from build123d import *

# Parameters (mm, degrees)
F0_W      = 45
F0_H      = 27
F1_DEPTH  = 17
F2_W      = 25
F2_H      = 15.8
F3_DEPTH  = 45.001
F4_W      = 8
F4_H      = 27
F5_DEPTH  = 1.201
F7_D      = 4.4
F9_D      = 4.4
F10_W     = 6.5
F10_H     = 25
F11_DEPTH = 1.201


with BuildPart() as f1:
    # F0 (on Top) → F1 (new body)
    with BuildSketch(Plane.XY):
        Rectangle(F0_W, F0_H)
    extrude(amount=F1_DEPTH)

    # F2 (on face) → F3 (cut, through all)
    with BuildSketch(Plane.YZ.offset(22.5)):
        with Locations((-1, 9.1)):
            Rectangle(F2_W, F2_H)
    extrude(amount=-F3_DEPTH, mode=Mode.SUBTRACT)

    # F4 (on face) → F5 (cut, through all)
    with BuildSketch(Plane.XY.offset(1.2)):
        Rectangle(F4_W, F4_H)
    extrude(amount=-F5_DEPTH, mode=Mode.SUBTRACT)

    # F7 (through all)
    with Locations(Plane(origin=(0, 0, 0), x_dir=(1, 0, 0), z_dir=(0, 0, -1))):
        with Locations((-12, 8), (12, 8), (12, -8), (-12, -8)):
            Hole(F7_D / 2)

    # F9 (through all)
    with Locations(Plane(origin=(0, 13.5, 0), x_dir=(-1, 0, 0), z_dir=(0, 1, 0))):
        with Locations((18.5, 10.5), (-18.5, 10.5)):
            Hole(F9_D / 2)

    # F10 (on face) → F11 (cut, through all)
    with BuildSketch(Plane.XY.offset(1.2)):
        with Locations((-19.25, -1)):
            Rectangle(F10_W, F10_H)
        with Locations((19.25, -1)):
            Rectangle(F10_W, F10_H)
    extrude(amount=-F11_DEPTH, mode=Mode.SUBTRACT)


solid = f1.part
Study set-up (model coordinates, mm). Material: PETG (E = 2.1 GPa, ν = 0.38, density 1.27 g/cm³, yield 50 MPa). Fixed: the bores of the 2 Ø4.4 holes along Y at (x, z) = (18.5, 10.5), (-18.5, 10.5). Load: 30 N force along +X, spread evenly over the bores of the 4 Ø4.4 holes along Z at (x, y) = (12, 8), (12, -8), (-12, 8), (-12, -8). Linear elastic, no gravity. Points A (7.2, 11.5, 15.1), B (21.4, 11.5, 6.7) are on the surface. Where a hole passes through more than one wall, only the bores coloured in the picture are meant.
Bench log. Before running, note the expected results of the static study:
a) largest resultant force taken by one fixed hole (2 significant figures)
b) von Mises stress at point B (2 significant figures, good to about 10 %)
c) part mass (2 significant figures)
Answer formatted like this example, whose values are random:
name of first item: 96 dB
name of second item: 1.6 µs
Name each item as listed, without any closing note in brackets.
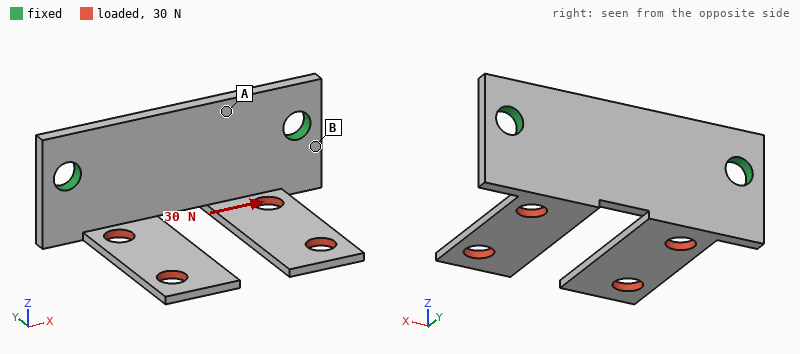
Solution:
largest resultant force taken by one fixed hole: 20 N
von Mises stress at point B: 6.0 MPa
part mass: 2.7 g
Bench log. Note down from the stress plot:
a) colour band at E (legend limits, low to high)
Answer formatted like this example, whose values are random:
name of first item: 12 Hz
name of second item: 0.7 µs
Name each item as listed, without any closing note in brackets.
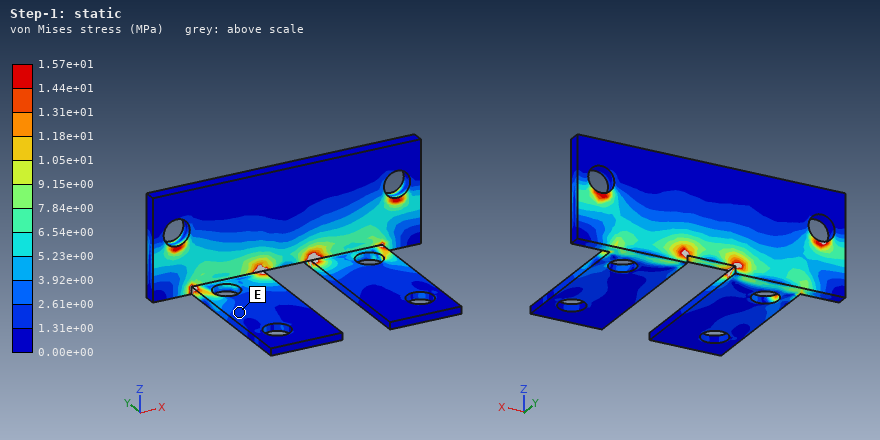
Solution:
colour band at E: 1.31e+00 to 2.61e+00 MPa
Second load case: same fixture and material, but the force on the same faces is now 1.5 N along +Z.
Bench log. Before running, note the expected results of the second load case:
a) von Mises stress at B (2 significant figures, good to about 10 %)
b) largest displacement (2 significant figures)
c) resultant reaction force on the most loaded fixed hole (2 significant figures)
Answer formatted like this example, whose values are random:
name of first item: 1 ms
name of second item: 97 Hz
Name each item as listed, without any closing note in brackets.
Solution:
von Mises stress at B: 0.62 MPa
largest displacement: 0.63 mm
resultant reaction force on the most loaded fixed hole: 0.79 N
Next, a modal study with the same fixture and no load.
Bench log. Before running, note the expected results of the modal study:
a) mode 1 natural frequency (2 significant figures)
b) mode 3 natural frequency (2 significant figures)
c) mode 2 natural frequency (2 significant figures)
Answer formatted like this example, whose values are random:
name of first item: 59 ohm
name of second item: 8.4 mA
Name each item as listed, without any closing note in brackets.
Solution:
mode 1 natural frequency: 330 Hz
mode 3 natural frequency: 840 Hz
mode 2 natural frequency: 340 Hz
